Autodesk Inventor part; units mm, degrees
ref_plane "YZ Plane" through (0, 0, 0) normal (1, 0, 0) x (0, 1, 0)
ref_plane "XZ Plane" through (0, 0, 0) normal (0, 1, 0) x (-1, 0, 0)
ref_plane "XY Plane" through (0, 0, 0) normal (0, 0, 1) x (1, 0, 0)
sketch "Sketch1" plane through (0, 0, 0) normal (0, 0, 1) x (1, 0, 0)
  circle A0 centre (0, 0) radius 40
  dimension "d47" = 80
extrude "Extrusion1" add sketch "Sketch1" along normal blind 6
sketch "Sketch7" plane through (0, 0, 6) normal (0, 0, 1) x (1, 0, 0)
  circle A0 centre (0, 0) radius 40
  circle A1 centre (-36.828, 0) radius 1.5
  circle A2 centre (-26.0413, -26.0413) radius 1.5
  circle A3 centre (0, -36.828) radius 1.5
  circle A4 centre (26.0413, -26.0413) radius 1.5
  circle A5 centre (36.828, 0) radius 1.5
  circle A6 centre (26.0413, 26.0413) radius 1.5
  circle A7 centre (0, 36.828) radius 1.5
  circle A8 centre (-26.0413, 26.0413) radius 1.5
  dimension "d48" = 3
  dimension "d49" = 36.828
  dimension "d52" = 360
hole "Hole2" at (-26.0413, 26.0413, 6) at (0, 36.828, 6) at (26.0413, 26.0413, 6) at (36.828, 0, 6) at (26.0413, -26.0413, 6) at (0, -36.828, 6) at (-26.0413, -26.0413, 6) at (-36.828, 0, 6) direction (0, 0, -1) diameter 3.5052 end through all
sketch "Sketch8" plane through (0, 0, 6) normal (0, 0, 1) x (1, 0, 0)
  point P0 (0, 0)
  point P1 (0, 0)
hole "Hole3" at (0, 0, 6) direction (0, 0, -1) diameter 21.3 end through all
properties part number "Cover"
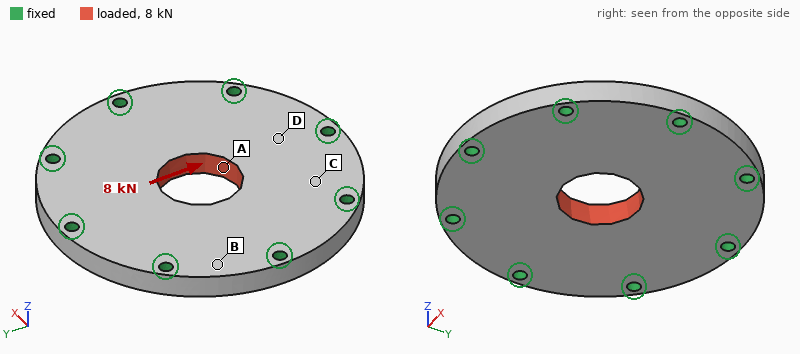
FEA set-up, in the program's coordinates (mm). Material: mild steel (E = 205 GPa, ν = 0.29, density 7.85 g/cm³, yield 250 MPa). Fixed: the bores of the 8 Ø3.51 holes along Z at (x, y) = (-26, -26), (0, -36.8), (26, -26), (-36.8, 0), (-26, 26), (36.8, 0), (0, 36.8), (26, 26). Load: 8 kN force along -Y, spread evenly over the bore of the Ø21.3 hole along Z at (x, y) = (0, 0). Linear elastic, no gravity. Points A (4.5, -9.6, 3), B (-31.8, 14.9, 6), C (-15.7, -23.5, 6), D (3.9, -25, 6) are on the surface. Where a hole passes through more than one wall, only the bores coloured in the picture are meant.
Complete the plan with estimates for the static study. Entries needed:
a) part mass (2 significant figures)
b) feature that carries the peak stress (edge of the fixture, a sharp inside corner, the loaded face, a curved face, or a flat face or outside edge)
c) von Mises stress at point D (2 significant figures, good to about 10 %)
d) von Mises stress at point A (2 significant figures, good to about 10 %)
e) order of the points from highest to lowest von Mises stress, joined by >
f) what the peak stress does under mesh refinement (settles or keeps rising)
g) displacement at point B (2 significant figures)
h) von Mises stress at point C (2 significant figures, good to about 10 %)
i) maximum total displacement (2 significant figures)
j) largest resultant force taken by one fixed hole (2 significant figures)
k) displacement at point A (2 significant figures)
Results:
220 g
edge of the fixture
16 MPa
22 MPa
A > D > C > B
keeps rising
0.50 µm
9.1 MPa
2.6 µm
1.6 kN
2.5 µm
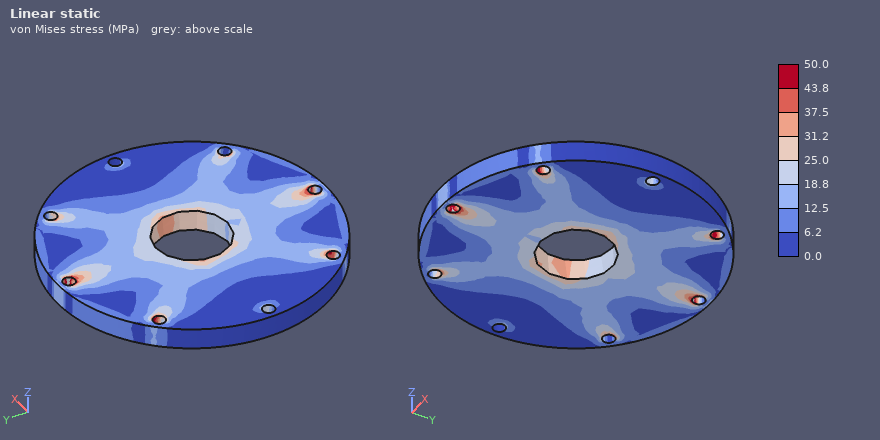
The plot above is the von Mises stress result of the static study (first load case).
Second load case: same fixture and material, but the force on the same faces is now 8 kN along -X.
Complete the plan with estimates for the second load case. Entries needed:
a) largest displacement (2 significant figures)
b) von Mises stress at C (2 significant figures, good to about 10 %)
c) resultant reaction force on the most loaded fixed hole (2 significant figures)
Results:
2.6 µm
12 MPa
1.6 kN
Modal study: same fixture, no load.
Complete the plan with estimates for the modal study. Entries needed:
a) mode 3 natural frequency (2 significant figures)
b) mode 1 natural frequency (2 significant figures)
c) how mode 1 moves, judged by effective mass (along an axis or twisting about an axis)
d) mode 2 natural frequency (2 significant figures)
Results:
16 kHz
9300 Hz
along Z
16 kHz
